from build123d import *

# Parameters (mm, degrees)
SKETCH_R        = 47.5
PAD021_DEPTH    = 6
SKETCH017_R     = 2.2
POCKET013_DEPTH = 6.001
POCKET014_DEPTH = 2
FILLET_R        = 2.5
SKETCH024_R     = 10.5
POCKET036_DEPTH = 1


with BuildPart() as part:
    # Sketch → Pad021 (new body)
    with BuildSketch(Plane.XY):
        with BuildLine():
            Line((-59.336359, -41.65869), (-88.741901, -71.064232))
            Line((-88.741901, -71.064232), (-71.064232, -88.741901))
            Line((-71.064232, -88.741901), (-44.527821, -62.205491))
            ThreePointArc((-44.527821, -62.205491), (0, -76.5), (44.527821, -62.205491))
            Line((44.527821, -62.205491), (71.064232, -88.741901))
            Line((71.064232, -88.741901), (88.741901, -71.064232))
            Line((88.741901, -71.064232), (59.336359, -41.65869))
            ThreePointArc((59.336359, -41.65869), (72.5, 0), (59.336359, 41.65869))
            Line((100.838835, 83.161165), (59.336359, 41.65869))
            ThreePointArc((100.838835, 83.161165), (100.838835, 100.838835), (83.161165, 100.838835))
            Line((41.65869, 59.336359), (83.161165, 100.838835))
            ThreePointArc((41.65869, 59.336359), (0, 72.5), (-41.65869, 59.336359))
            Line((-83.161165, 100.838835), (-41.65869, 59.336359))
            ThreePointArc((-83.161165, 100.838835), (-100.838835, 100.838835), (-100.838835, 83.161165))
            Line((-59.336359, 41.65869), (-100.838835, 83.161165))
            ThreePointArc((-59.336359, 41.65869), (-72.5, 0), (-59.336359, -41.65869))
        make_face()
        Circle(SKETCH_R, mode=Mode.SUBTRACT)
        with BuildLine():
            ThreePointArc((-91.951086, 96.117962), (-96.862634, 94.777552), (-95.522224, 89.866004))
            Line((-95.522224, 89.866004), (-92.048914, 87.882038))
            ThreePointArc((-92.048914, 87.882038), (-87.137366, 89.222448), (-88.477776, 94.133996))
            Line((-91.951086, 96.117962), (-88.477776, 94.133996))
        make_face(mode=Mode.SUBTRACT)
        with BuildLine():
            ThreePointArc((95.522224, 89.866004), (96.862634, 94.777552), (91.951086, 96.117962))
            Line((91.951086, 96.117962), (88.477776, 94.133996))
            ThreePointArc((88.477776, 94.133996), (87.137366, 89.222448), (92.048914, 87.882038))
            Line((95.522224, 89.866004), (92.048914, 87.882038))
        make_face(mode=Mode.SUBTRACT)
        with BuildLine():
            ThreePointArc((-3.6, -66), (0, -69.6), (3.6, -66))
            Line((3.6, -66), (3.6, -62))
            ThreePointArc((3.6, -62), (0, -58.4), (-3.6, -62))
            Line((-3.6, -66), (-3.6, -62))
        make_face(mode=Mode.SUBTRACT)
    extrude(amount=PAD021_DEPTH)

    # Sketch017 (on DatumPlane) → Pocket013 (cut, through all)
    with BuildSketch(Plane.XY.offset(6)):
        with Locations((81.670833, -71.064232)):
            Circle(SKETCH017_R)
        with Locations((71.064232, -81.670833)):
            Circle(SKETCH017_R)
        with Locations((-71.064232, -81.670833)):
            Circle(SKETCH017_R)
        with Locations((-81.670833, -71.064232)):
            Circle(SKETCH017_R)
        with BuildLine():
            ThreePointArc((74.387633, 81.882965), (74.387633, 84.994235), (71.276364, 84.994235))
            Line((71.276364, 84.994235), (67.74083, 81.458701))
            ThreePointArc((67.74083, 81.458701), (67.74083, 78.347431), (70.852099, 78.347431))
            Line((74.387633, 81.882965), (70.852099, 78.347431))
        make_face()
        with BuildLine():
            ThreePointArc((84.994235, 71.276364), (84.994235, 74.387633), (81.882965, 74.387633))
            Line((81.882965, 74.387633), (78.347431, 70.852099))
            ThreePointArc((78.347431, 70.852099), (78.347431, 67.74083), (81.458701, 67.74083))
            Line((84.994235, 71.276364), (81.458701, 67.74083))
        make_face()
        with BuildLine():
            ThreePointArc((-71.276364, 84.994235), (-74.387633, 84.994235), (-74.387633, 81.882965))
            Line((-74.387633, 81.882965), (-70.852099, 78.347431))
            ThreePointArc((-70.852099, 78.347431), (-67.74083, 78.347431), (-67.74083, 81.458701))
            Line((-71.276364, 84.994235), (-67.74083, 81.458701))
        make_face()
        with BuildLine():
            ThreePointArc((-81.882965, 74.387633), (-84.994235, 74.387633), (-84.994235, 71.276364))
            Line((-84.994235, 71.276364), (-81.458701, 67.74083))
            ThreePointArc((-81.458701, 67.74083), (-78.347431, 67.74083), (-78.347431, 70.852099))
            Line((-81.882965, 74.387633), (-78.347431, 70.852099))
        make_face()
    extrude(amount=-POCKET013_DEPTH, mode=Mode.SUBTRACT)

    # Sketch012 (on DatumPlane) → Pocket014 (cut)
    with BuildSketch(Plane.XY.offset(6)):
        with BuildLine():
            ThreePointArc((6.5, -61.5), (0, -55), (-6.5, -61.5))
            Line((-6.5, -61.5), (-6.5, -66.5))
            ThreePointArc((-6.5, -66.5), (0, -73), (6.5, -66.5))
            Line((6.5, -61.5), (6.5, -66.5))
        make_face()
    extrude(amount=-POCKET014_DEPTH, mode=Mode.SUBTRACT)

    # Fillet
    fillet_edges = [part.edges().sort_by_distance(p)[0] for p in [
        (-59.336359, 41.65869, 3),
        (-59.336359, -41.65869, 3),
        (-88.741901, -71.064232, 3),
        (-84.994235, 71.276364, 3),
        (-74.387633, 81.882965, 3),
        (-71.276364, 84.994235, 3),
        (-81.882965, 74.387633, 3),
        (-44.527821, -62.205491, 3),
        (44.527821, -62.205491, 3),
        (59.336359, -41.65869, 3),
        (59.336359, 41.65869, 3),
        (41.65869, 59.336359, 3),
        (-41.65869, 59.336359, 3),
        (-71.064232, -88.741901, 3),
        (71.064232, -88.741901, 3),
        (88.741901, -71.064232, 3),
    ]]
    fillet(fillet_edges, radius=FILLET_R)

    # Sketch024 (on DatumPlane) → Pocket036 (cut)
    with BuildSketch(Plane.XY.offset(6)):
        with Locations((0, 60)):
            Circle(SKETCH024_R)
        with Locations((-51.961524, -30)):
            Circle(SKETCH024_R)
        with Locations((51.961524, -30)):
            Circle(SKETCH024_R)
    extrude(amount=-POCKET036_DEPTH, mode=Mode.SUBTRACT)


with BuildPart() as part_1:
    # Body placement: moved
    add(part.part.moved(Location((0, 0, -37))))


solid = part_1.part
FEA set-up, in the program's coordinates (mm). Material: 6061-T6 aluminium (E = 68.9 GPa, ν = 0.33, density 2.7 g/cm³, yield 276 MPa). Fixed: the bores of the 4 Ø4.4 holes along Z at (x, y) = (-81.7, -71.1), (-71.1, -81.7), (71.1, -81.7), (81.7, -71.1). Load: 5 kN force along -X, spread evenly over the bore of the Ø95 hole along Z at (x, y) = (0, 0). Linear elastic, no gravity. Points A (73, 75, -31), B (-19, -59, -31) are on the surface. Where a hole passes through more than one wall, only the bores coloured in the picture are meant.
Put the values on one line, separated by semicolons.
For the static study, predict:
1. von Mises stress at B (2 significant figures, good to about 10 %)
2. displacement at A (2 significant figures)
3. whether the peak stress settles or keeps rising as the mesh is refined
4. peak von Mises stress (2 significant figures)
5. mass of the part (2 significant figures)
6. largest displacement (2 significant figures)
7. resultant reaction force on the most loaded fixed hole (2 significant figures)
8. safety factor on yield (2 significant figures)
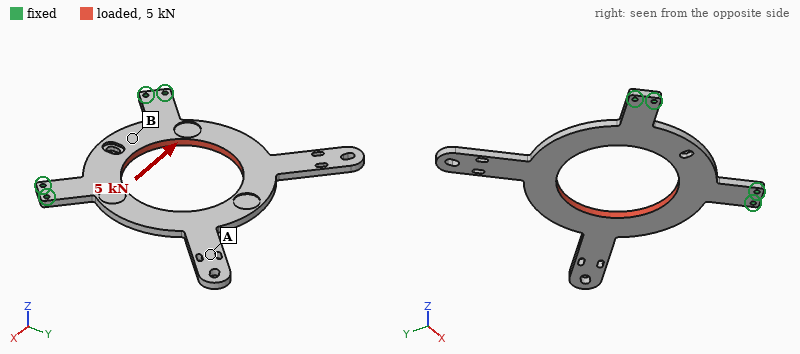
24 MPa; 0.31 mm; settles; 200 MPa; 240 g; 0.35 mm; 2.7 kN; 1.4
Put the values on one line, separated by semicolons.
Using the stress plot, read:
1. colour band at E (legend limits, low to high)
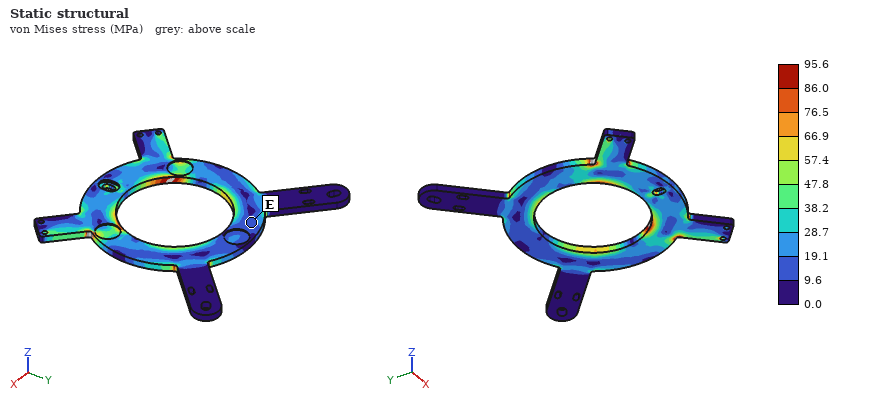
9.6 to 19.1 MPa
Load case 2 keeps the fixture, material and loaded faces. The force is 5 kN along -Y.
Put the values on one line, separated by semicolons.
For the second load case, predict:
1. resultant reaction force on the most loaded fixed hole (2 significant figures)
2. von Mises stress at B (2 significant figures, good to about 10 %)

2.6 kN; 8.4 MPa
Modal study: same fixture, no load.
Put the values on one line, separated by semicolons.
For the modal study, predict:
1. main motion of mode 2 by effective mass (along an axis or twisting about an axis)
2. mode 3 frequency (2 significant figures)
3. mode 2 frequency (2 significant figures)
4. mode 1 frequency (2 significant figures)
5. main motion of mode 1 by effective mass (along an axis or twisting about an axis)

twisting about Y; 670 Hz; 260 Hz; 120 Hz; along Z
